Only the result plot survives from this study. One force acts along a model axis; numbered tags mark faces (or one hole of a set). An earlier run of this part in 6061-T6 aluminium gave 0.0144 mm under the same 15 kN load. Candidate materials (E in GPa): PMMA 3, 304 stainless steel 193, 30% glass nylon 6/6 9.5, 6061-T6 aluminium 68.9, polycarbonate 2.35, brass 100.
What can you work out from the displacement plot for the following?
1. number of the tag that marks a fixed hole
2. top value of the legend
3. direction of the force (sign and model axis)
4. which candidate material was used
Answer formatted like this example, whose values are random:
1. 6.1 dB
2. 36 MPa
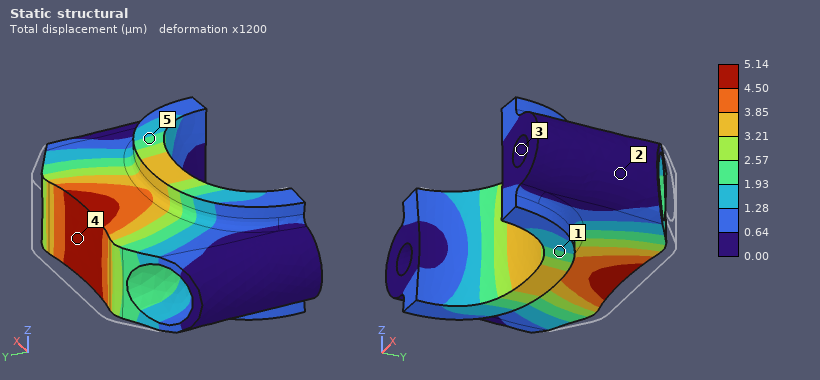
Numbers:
1. 3
2. 5.14 µm
3. -Y
4. 304 stainless steel
